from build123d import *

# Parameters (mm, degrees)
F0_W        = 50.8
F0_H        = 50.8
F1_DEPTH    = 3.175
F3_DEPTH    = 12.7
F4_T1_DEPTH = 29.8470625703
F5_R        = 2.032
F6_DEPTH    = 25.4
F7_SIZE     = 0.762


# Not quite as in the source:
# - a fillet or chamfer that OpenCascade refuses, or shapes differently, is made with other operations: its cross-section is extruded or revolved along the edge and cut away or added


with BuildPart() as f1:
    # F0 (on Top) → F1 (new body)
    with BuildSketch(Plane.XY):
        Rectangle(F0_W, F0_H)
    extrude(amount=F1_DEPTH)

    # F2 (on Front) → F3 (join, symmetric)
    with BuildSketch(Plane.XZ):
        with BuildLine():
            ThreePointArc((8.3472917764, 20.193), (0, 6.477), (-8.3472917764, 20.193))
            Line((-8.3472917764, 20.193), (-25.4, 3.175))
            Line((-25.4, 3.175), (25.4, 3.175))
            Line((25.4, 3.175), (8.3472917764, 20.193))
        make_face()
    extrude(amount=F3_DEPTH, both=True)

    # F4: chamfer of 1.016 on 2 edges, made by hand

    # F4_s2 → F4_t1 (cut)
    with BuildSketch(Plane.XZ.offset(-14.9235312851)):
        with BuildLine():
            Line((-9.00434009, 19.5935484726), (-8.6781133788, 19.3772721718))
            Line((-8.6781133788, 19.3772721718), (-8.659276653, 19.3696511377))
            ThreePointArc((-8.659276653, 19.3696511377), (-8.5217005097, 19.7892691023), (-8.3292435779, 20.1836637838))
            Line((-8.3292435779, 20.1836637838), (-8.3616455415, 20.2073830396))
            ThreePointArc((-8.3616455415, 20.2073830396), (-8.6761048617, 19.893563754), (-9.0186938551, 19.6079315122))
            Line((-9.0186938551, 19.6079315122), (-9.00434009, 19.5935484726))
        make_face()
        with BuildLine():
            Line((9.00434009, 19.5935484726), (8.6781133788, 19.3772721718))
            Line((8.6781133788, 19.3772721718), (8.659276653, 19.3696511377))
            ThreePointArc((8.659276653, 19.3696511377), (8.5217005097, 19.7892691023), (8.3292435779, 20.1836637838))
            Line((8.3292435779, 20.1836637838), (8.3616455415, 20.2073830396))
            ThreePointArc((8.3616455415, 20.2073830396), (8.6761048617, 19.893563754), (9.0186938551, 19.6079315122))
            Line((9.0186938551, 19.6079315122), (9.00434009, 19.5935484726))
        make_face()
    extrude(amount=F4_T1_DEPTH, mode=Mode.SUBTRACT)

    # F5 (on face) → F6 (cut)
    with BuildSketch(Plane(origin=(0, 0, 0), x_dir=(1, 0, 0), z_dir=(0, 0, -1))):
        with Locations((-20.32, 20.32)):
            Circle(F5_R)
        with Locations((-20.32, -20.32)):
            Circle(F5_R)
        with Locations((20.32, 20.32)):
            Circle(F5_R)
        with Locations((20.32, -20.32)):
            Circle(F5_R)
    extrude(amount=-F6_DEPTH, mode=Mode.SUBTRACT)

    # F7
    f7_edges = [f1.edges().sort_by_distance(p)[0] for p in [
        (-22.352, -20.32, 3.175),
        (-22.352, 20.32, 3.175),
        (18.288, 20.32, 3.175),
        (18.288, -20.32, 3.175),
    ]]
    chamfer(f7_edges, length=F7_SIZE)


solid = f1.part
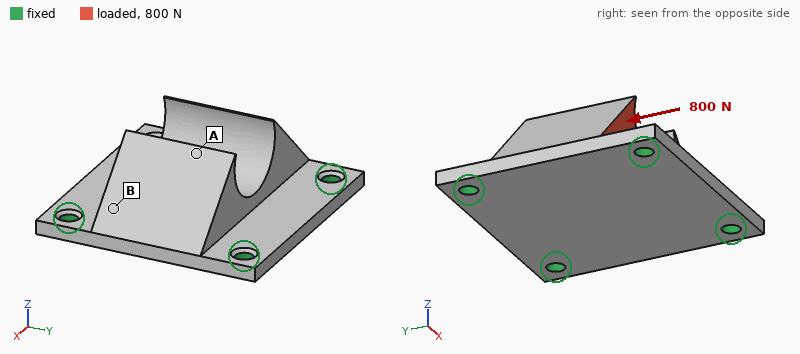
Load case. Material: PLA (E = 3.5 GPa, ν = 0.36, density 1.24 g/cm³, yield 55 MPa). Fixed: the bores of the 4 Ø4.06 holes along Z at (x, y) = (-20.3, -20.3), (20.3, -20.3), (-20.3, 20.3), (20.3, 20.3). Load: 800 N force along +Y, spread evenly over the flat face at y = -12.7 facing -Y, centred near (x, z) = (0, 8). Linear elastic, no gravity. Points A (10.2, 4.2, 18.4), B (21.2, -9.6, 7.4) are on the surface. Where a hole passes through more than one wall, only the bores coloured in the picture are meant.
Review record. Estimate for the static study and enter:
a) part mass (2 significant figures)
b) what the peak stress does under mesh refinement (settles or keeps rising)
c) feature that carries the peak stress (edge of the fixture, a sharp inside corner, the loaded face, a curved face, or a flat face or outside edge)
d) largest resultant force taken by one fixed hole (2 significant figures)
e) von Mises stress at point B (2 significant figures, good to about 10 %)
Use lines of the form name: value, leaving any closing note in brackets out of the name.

part mass: 21 g
what the peak stress does under mesh refinement: keeps rising
feature that carries the peak stress: edge of the fixture
largest resultant force taken by one fixed hole: 230 N
von Mises stress at point B: 3.1 MPa
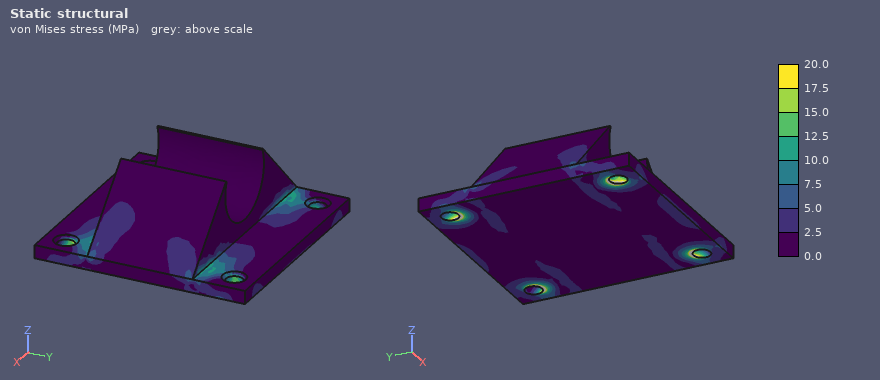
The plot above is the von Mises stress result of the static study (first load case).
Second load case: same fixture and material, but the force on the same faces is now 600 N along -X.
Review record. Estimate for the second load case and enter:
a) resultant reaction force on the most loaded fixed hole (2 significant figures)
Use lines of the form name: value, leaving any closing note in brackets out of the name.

resultant reaction force on the most loaded fixed hole: 210 N
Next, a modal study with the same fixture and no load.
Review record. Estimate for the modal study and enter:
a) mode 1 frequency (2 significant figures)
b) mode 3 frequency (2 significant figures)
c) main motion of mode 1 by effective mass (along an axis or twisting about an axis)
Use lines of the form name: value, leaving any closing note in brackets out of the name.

mode 1 frequency: 2500 Hz
mode 3 frequency: 4200 Hz
main motion of mode 1 by effective mass: along Z
